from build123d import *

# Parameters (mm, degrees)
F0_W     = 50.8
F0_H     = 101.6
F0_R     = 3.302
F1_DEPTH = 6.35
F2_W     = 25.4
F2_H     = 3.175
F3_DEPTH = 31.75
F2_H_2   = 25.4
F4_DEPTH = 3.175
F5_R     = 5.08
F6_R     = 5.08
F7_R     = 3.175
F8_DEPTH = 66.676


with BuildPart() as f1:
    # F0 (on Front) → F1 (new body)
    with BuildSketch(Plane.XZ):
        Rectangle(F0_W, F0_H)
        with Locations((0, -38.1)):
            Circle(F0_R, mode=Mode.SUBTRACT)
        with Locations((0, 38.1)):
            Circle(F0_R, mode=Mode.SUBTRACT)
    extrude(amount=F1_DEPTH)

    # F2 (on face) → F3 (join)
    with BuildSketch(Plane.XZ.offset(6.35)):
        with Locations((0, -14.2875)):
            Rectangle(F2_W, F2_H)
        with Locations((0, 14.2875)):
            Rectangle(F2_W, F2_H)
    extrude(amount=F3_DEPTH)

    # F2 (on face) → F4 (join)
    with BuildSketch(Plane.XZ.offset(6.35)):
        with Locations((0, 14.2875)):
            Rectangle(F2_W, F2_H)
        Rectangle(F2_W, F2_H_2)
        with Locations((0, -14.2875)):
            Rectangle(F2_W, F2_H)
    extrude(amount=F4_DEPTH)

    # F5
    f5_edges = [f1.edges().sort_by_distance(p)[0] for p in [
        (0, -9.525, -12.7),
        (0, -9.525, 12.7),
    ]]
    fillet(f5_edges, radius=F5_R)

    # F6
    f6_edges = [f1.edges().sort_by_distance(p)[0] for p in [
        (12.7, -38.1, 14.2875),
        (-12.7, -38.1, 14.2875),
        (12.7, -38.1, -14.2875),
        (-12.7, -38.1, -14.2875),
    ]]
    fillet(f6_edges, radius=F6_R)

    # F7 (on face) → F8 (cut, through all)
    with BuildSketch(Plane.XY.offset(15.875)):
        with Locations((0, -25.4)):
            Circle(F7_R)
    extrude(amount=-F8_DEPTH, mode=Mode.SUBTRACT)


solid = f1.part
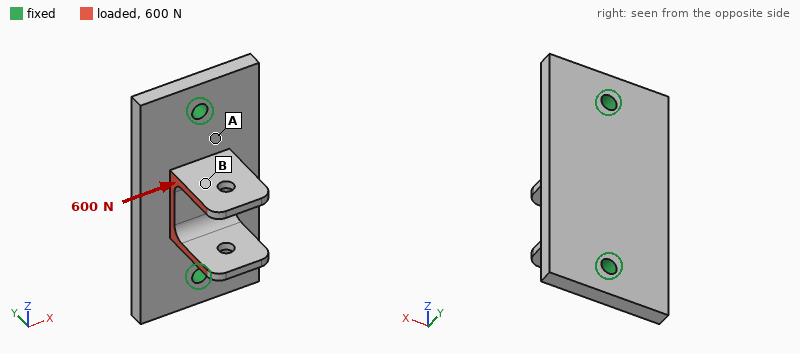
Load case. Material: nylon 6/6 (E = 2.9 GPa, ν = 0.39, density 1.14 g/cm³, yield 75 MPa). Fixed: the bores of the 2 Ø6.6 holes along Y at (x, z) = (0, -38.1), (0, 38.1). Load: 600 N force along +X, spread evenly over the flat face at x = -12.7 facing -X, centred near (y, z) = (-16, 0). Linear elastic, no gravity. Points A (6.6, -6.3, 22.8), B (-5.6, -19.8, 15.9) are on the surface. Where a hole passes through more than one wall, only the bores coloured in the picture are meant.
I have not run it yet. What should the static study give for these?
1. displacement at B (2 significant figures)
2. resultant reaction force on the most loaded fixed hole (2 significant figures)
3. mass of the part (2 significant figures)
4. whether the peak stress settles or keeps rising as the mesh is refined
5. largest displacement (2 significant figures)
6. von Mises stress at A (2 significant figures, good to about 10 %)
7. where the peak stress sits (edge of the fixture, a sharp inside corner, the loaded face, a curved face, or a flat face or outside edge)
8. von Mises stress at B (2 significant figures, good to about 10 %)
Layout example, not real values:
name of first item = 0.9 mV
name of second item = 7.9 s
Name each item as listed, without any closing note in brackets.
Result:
displacement at B = 0.42 mm
resultant reaction force on the most loaded fixed hole = 300 N
mass of the part = 45 g
whether the peak stress settles or keeps rising as the mesh is refined = keeps rising
largest displacement = 0.82 mm
von Mises stress at A = 8.4 MPa
where the peak stress sits = edge of the fixture
von Mises stress at B = 3.8 MPa
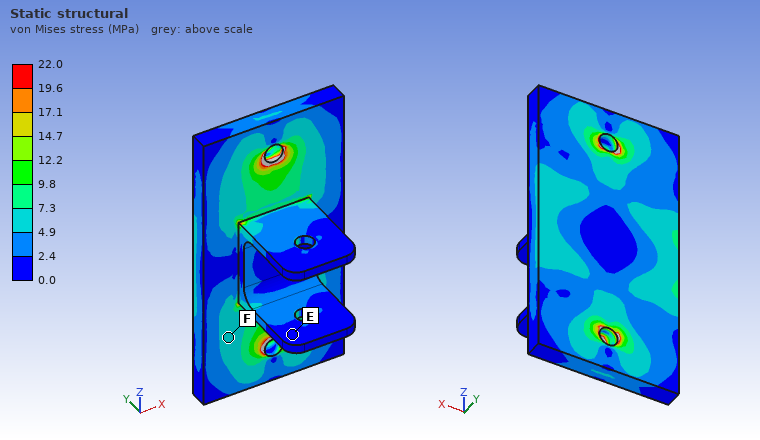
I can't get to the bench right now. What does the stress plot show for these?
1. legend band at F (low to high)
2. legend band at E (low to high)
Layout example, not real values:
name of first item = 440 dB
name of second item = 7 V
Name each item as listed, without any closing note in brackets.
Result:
legend band at F = 4.9 to 7.3 MPa
legend band at E = 0.0 to 2.4 MPa
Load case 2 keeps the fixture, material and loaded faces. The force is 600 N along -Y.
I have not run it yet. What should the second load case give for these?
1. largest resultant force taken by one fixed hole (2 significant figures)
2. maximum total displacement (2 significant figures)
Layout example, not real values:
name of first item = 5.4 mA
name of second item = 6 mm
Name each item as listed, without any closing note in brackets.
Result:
largest resultant force taken by one fixed hole = 320 N
maximum total displacement = 0.90 mm
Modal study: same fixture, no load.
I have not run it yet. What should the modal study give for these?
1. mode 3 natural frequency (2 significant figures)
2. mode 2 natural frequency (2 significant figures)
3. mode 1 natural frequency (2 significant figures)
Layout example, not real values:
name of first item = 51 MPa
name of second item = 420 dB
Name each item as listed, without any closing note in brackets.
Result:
mode 3 natural frequency = 1100 Hz
mode 2 natural frequency = 1100 Hz
mode 1 natural frequency = 1100 Hz
